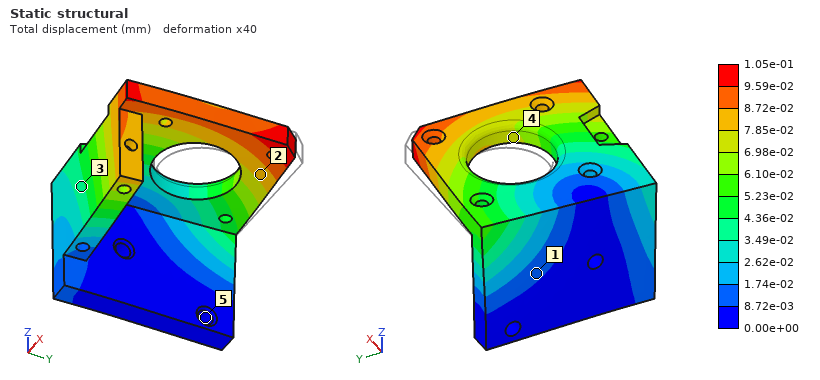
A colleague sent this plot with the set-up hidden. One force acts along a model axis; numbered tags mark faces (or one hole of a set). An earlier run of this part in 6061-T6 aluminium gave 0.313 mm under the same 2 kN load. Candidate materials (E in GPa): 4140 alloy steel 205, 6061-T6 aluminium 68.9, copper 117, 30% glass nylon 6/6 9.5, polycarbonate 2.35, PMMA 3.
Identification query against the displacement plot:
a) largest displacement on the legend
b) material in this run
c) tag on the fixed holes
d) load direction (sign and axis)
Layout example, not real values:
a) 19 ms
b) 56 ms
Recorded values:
a) 1.05e-01 mm
b) 4140 alloy steel
c) 5
d) -Y
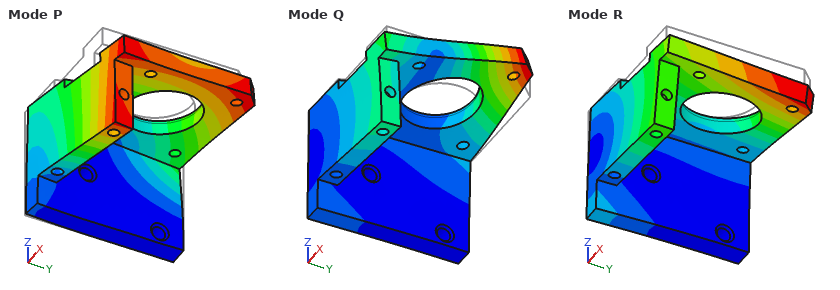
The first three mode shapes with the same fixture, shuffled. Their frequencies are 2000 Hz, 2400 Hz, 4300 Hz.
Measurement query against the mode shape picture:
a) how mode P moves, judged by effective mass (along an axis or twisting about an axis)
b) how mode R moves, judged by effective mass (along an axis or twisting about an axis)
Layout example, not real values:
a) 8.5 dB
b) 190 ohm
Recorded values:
a) along Y
b) along Z
